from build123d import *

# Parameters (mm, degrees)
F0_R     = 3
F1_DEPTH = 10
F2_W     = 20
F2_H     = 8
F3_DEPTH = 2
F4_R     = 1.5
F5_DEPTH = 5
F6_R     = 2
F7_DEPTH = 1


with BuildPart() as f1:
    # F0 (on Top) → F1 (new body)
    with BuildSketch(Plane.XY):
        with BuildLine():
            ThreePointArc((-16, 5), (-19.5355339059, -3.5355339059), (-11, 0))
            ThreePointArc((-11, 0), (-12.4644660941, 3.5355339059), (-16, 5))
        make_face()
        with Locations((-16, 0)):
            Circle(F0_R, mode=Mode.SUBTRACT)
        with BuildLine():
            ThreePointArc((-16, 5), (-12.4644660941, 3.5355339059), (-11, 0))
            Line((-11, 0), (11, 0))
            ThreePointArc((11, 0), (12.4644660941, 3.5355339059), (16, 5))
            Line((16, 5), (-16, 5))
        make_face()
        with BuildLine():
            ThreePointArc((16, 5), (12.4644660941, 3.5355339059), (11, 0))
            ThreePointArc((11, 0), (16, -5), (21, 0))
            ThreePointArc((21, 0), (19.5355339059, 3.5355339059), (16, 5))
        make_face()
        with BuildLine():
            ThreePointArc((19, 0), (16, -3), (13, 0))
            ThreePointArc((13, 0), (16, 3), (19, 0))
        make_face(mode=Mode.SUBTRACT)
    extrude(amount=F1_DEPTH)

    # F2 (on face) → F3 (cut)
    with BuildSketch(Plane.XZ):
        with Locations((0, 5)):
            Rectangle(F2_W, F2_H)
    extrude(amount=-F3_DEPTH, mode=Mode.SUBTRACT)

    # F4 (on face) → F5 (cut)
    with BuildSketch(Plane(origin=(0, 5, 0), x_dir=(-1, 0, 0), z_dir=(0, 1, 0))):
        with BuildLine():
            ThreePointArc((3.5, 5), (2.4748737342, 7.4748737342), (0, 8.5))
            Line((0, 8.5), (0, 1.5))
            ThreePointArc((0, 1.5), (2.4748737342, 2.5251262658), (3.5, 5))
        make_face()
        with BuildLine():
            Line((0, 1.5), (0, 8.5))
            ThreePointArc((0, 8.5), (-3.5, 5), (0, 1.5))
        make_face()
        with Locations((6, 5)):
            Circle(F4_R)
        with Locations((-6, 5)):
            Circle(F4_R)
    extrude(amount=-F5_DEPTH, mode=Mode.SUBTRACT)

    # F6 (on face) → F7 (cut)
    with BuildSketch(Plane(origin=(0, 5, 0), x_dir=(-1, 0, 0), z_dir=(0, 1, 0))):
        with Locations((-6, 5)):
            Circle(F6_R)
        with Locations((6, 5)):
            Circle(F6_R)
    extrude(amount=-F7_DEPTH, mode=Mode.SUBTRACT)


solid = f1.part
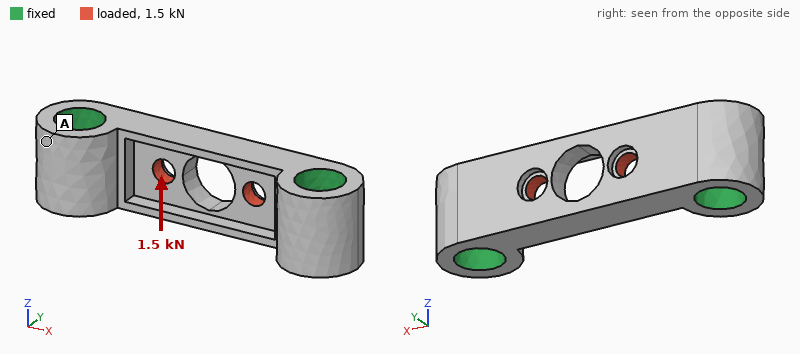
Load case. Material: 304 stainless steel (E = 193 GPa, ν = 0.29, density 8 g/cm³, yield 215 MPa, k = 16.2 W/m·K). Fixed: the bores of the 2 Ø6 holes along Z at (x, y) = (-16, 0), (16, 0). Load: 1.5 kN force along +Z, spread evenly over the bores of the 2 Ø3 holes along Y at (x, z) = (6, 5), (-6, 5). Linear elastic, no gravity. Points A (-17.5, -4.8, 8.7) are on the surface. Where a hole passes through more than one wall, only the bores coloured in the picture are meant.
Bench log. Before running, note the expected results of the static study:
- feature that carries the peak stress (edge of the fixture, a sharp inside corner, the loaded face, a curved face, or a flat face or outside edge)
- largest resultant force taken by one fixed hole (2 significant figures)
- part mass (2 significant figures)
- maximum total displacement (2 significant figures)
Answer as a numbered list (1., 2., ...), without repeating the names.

1. the loaded face
2. 750 N
3. 14 g
4. 7.5 µm
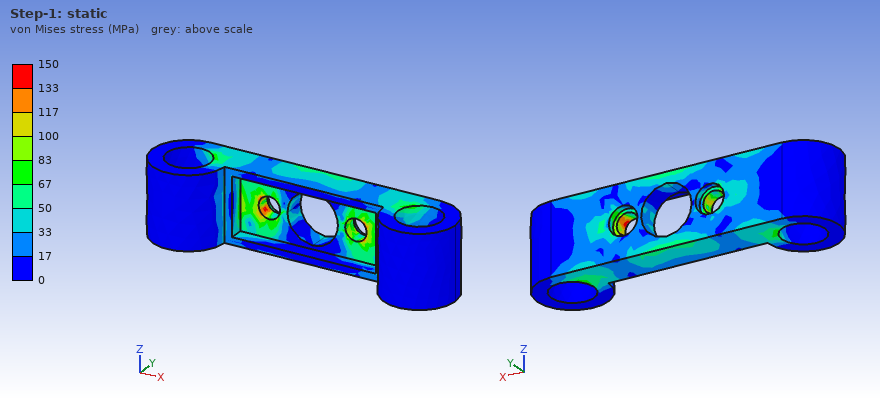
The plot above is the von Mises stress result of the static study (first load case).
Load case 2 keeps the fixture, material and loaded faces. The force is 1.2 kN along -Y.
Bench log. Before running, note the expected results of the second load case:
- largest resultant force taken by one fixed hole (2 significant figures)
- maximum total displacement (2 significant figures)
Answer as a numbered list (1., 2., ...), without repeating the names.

1. 610 N
2. 10 µm
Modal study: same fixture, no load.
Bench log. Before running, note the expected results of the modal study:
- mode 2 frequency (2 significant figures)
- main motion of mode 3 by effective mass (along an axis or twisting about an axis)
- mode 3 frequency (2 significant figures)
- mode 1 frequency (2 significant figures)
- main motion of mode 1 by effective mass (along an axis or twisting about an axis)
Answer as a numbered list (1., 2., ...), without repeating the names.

1. 36 kHz
2. along Z
3. 46 kHz
4. 33 kHz
5. along Y
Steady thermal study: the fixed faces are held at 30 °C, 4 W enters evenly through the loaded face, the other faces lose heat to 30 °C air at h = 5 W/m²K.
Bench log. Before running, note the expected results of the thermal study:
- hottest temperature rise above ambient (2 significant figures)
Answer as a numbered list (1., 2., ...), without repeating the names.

1. 37 K
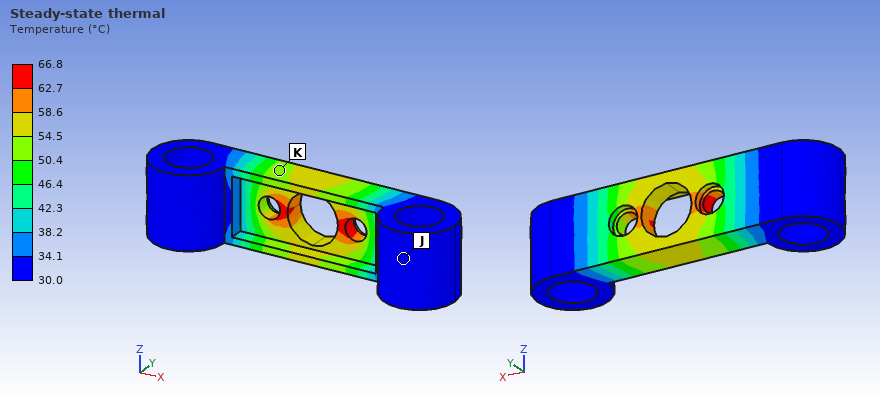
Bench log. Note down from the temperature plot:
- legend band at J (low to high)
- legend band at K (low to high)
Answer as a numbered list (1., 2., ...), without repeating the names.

1. 30.0 to 34.1 °C
2. 50.4 to 54.5 °C
